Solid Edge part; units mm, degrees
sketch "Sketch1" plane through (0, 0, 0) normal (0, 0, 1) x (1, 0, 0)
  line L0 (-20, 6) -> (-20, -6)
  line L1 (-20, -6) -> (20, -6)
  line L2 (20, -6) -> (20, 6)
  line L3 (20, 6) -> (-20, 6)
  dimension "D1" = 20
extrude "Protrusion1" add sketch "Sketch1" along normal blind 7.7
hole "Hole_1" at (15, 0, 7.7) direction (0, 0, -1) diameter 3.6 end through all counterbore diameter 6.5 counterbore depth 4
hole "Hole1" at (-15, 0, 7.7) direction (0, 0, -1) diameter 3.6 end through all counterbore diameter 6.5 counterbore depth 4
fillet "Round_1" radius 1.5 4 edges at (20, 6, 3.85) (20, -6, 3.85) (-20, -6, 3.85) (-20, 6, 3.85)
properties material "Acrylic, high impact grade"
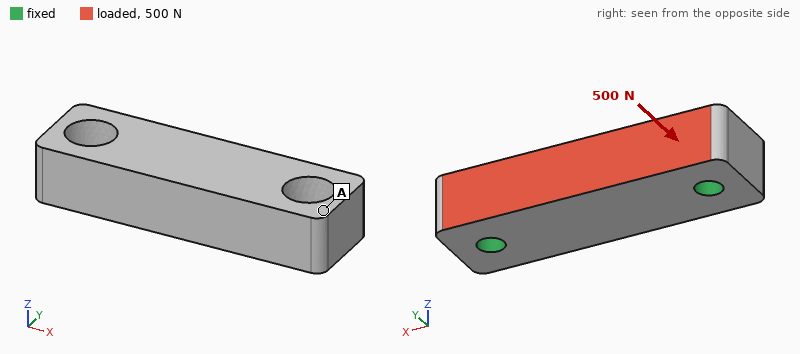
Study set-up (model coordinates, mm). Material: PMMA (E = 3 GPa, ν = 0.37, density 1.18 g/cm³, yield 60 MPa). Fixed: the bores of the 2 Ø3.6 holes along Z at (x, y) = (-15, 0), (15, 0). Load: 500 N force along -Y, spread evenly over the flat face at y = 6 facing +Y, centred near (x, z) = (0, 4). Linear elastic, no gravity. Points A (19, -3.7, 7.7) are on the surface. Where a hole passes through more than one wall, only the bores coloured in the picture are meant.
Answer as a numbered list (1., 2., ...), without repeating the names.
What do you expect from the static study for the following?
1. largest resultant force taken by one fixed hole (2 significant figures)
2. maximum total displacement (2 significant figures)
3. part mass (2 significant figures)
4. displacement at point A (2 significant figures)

1. 250 N
2. 78 µm
3. 3.9 g
4. 21 µm
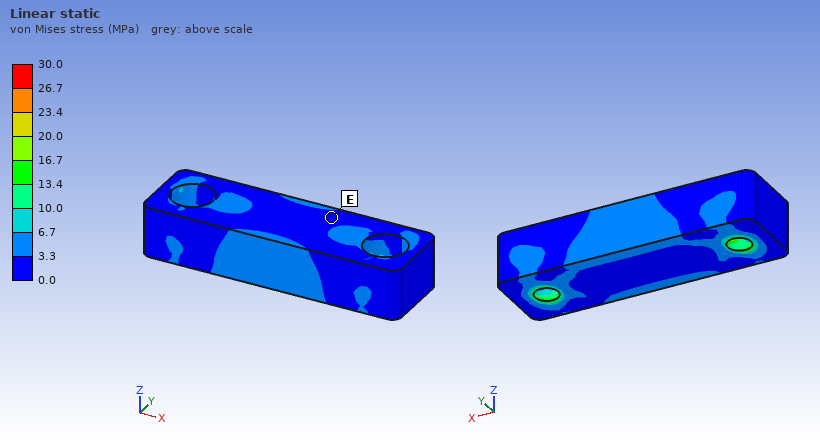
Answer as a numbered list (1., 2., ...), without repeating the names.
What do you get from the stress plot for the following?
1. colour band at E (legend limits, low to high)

1. 0.0 to 3.3 MPa
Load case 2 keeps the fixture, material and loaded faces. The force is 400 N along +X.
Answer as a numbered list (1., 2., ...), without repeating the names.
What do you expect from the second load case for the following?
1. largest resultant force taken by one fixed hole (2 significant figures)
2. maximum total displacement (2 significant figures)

1. 210 N
2. 22 µm
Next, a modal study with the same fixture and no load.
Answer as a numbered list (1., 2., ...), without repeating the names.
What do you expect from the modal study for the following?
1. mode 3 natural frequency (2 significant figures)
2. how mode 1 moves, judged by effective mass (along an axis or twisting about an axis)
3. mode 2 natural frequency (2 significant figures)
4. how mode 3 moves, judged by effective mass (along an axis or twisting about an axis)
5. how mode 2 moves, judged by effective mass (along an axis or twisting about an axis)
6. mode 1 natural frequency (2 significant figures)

1. 10 kHz
2. along Y
3. 8000 Hz
4. along Y
5. along Z
6. 7500 Hz
